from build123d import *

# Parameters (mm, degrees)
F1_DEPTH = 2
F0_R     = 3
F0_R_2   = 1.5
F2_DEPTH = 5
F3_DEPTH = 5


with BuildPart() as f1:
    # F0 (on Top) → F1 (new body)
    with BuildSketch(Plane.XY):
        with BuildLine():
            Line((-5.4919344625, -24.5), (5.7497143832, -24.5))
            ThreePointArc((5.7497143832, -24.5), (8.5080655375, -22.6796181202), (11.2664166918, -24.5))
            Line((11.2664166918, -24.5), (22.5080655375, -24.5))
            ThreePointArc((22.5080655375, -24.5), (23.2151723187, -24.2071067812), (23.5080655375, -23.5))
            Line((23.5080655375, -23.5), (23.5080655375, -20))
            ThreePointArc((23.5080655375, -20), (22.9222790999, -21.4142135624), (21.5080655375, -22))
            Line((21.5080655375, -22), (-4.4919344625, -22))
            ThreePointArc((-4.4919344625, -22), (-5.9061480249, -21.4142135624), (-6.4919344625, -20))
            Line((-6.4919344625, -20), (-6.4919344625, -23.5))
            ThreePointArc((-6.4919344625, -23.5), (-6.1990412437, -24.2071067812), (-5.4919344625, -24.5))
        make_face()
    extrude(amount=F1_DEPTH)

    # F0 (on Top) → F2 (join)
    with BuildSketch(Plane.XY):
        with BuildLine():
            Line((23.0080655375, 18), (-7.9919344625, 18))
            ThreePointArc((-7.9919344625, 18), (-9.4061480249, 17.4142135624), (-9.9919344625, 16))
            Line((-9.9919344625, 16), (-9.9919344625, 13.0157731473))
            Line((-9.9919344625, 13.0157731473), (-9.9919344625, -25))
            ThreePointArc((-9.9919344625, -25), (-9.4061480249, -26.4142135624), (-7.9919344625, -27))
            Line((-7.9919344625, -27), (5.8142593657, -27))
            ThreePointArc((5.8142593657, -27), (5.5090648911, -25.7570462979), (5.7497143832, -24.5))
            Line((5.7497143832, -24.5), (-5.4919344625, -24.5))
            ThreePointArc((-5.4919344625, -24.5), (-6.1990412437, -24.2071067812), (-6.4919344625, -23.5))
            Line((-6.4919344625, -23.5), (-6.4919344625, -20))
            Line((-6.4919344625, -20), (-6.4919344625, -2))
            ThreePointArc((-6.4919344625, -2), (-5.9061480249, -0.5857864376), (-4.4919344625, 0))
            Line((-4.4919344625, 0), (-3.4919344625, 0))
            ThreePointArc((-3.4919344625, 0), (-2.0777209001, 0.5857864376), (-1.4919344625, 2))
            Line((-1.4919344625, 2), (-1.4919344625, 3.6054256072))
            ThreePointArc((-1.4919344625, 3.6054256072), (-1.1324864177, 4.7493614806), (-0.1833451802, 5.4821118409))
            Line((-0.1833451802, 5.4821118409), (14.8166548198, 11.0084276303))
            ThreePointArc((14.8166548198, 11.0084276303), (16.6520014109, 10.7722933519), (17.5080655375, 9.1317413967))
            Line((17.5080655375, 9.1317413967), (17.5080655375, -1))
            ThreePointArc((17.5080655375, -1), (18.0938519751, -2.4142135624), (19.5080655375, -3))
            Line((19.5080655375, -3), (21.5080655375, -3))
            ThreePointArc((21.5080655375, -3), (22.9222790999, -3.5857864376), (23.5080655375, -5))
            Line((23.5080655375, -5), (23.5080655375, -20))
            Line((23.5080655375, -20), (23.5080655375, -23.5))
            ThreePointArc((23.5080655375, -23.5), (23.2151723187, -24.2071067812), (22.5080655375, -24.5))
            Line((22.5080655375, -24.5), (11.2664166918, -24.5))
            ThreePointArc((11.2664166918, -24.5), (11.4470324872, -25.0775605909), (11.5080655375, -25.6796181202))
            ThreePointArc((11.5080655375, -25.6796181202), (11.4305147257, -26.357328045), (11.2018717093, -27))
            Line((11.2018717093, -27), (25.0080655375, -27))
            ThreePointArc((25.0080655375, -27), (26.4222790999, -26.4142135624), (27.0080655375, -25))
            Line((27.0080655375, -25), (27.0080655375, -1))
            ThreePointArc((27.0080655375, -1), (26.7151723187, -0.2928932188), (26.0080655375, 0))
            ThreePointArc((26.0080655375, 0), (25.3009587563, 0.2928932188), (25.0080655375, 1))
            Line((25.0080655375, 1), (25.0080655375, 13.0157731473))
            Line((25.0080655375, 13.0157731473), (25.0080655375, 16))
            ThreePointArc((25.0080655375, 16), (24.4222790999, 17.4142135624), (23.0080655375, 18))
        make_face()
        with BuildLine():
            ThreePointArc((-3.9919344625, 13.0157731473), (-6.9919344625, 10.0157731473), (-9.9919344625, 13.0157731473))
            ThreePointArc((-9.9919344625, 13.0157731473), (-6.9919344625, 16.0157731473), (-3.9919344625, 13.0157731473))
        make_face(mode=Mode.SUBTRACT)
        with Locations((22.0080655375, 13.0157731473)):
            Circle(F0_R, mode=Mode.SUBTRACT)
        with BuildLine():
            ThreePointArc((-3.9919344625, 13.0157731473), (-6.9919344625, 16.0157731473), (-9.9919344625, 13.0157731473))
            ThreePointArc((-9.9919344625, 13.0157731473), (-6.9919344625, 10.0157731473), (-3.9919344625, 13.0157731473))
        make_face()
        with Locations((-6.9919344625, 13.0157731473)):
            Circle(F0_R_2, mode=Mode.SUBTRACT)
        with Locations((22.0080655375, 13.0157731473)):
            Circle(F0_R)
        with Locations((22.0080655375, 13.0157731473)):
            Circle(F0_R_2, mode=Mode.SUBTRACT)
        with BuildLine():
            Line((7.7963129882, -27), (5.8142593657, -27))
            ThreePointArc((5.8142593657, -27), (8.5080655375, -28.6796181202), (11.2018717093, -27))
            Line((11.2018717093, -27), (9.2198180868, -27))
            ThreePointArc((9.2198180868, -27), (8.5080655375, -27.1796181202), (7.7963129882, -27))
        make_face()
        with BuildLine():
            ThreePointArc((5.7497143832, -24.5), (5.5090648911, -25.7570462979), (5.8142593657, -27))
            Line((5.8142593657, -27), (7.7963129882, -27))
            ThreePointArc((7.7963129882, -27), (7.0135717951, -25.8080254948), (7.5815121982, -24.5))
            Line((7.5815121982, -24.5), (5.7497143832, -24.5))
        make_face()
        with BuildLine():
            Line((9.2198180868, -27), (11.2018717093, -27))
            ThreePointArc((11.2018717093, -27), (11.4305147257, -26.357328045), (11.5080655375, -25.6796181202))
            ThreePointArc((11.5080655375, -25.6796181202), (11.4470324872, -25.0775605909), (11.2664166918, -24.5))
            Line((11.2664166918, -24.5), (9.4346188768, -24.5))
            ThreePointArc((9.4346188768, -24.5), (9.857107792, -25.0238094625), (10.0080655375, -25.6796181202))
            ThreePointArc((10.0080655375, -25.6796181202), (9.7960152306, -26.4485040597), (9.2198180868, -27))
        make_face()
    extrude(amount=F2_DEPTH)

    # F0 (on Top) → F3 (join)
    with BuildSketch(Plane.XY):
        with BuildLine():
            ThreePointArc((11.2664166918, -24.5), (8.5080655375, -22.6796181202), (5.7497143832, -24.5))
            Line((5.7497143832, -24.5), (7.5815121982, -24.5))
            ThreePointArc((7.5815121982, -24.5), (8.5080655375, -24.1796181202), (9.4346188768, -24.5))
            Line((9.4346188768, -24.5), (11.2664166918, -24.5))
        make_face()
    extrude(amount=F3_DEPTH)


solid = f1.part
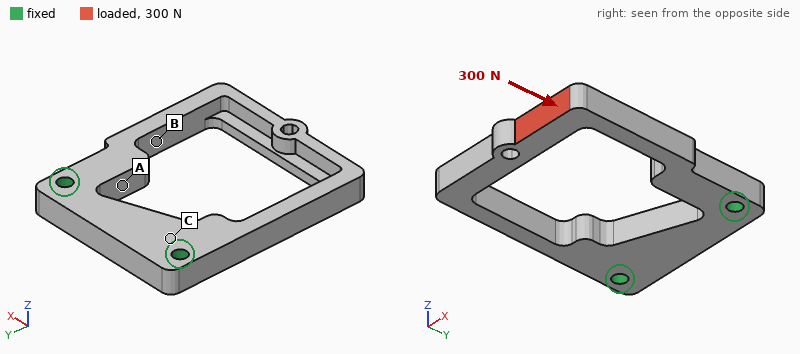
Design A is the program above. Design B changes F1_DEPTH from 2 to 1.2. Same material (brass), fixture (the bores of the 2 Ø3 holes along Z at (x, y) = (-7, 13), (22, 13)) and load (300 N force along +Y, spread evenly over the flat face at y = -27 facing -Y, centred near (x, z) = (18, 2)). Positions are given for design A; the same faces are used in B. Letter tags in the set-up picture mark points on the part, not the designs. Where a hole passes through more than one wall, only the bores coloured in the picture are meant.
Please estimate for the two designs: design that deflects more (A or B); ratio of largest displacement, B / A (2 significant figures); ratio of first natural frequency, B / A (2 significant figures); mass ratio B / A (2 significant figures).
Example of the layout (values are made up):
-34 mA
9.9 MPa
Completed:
B
1.2
1.0
0.99
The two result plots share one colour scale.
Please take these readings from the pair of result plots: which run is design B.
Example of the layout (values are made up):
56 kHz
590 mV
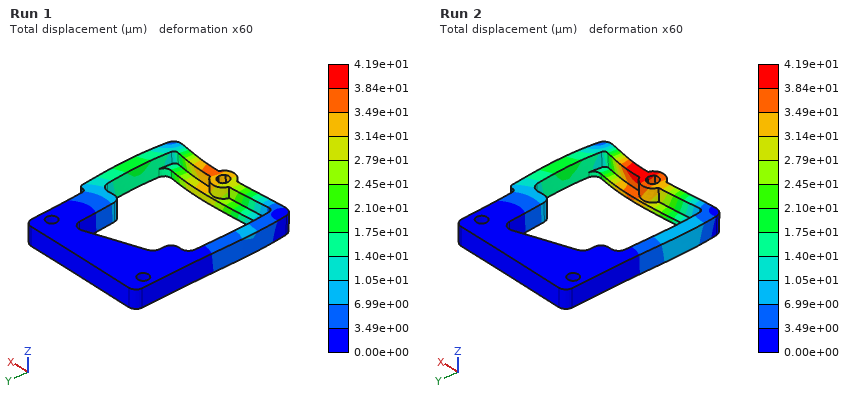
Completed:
Run 2
